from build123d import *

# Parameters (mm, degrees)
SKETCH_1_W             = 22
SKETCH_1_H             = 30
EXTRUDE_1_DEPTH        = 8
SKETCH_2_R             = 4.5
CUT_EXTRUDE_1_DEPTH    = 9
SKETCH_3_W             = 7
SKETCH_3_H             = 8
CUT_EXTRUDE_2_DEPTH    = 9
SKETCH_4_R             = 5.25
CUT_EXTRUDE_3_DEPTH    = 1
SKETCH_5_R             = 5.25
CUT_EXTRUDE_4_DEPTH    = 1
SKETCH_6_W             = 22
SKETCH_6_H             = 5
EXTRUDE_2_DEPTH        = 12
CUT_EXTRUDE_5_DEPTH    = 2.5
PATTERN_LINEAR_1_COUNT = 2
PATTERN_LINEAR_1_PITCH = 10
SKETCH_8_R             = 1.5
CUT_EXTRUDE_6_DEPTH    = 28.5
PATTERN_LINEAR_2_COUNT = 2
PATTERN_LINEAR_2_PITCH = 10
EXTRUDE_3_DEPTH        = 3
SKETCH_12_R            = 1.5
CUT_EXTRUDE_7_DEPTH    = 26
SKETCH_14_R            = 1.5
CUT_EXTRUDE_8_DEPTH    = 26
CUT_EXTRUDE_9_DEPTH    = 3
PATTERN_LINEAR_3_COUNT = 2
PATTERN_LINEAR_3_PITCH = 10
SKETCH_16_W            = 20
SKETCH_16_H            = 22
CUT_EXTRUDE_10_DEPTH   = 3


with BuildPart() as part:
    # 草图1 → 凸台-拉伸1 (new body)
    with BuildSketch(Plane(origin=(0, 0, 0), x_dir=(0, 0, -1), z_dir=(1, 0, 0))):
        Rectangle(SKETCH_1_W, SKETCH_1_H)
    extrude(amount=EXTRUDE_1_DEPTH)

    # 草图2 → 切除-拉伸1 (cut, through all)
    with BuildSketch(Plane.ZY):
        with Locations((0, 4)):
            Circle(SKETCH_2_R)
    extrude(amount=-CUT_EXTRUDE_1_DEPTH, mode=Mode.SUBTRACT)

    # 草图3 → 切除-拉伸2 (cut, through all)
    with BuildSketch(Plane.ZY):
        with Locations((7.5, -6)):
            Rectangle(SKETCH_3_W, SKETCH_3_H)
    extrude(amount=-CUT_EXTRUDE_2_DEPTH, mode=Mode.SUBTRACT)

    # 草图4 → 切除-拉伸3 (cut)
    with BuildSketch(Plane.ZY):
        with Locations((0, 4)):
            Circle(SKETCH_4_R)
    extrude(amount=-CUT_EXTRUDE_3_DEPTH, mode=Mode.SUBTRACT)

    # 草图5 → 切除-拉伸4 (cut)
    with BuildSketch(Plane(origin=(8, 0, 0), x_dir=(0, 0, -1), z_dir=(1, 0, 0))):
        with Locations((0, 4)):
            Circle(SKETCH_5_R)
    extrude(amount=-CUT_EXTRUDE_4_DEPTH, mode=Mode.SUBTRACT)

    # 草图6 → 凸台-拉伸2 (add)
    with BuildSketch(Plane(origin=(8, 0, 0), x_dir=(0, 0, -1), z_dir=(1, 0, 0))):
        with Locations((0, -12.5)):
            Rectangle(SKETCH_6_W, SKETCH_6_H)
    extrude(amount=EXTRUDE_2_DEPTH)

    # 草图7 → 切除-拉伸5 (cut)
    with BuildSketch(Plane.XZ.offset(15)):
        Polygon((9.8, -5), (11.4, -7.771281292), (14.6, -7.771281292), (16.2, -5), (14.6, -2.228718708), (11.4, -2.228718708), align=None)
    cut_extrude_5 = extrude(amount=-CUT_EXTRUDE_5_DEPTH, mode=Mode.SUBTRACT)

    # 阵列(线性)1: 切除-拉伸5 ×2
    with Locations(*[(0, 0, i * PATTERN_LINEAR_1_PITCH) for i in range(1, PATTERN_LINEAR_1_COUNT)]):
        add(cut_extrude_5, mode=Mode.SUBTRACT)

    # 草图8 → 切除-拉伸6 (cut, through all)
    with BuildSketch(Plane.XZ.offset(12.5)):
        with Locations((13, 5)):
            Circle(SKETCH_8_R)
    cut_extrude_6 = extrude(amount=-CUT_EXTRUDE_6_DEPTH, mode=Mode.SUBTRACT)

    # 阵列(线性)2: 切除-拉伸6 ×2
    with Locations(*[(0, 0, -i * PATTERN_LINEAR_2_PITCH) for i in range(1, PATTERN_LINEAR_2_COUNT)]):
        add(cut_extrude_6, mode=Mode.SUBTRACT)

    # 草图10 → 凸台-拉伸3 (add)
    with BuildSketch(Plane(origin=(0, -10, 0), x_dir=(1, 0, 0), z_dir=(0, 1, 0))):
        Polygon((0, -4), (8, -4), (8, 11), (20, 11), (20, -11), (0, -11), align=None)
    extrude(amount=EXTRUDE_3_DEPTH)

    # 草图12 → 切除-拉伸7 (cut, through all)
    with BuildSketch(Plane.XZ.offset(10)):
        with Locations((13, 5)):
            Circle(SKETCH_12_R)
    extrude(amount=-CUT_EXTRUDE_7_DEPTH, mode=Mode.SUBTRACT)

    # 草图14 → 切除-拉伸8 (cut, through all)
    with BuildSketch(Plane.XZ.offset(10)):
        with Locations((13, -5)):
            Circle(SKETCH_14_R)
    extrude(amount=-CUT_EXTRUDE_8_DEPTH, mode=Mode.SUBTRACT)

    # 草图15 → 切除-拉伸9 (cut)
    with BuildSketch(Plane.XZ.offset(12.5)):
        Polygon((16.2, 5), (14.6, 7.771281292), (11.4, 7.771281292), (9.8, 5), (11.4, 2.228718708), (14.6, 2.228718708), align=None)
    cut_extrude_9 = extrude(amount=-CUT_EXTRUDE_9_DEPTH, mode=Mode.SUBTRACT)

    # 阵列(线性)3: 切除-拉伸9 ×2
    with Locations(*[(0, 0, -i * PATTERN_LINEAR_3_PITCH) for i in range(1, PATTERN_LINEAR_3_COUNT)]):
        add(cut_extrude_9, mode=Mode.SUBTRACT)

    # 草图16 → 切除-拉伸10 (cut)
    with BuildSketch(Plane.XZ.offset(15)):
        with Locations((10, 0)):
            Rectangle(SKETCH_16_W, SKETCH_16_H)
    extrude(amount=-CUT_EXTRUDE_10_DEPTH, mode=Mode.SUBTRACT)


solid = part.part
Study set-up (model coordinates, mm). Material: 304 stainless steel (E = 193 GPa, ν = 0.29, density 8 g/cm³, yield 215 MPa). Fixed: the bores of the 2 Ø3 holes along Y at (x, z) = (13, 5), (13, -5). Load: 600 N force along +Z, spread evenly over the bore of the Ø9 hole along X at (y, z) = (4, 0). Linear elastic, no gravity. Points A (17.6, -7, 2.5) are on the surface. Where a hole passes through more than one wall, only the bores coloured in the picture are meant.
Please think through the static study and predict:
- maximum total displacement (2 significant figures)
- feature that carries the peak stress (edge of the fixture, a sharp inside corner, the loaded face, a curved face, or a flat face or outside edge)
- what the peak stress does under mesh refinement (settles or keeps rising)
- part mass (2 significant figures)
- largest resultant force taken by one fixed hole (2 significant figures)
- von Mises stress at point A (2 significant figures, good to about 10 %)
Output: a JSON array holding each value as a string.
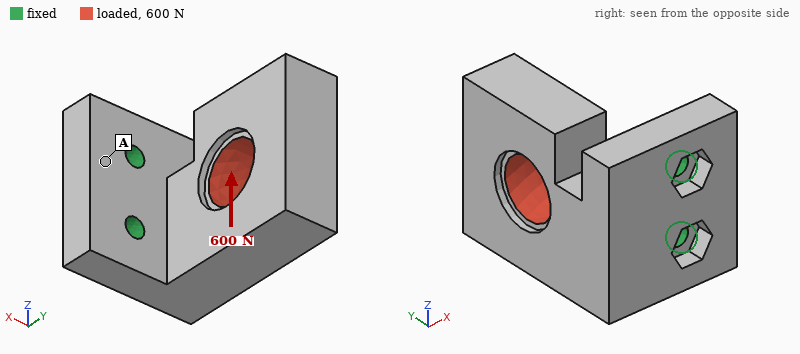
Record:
["27 µm", "edge of the fixture", "keeps rising", "41 g", "810 N", "20 MPa"]
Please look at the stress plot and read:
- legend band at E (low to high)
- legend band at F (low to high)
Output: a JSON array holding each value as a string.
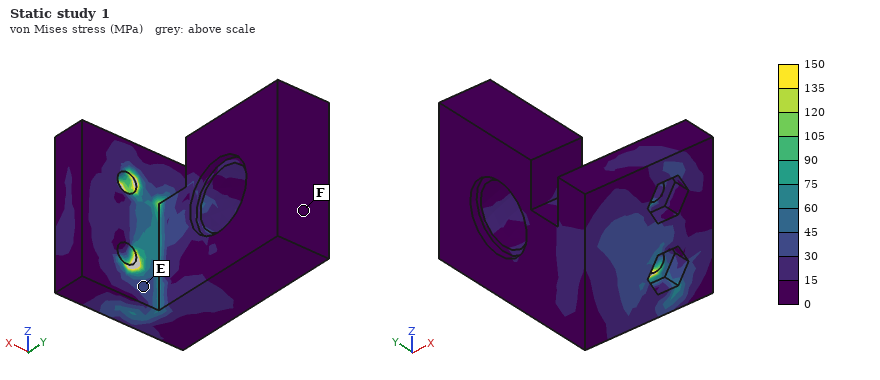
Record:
["30 to 45 MPa", "0 to 15 MPa"]
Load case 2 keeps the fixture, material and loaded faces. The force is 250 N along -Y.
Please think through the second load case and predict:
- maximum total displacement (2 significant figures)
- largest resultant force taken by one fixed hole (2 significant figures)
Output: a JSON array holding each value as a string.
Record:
["15 µm", "130 N"]
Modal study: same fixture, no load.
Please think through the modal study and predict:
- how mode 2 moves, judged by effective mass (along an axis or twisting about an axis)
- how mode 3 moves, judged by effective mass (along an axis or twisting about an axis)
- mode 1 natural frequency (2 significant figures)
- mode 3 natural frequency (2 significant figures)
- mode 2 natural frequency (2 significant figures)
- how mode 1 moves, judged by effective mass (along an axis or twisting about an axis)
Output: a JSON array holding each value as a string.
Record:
["along Z", "along Y", "3000 Hz", "12 kHz", "5300 Hz", "along X"]
